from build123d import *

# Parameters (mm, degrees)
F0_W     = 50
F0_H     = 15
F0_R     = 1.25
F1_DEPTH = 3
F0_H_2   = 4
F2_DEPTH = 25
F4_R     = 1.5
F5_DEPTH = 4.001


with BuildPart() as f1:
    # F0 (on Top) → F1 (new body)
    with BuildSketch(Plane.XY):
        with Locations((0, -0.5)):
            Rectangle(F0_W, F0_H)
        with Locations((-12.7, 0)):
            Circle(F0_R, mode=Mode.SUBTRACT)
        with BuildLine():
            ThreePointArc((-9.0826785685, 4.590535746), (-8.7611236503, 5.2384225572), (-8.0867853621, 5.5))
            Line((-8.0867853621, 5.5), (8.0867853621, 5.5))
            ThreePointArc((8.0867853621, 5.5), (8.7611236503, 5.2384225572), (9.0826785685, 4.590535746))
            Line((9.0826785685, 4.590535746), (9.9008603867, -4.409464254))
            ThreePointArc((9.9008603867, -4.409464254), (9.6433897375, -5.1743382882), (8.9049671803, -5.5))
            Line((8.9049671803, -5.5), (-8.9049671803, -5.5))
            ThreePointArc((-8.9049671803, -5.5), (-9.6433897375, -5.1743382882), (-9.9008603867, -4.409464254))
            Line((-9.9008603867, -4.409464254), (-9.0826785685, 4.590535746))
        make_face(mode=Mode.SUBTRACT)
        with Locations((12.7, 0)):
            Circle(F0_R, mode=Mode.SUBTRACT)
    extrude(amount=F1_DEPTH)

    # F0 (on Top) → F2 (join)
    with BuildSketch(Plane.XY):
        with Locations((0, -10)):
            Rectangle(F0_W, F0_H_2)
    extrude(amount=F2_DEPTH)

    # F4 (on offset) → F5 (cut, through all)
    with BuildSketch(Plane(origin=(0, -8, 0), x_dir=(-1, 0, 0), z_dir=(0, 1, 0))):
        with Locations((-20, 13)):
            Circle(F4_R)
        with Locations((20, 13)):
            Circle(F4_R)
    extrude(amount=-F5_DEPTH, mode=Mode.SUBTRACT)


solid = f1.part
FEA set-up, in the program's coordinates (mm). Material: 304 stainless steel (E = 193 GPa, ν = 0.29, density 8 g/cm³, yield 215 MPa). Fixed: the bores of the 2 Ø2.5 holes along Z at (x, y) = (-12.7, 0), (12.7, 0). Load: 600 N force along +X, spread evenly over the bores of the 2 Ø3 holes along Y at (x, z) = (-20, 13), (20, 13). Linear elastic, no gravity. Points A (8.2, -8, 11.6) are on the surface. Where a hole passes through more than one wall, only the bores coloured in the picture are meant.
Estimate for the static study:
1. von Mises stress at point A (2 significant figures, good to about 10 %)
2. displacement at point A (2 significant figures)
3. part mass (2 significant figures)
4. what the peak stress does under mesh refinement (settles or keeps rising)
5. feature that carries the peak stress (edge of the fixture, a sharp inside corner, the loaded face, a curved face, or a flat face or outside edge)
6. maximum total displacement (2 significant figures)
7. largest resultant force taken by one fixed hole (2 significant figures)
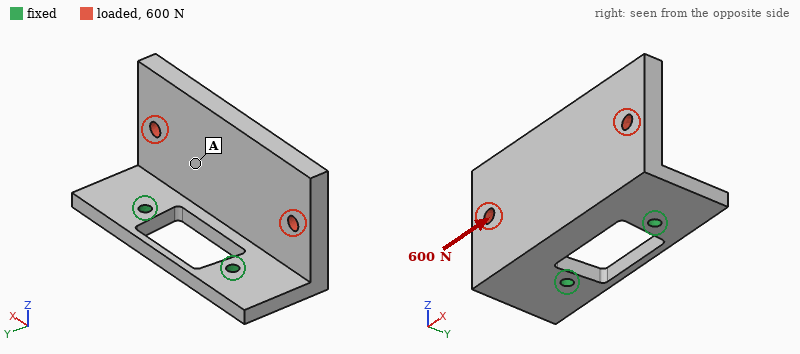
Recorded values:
13 MPa
9.0 µm
52 g
keeps rising
edge of the fixture
19 µm
400 N
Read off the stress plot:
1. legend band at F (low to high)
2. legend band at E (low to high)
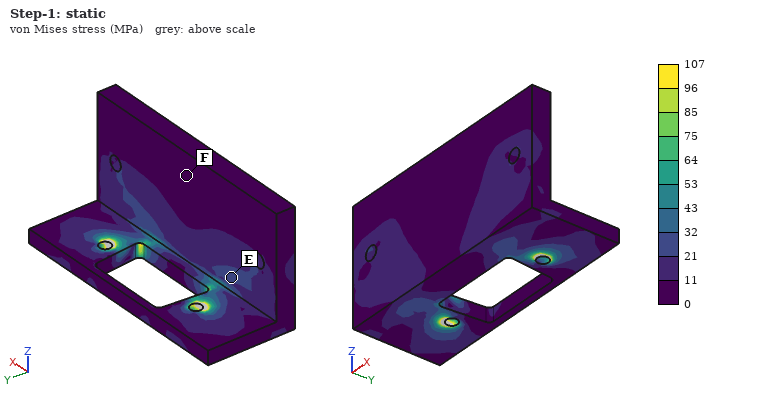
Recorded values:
0 to 11 MPa
21 to 32 MPa
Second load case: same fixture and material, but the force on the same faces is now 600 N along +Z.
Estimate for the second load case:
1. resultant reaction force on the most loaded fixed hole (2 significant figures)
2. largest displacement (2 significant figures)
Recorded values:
300 N
71 µm
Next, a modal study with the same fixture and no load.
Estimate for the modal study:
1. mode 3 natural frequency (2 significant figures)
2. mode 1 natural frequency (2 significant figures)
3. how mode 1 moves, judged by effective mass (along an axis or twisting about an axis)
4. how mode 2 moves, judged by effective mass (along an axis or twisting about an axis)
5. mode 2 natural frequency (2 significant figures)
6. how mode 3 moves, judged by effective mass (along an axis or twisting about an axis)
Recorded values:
6600 Hz
1900 Hz
along Y
along X
4300 Hz
along X
